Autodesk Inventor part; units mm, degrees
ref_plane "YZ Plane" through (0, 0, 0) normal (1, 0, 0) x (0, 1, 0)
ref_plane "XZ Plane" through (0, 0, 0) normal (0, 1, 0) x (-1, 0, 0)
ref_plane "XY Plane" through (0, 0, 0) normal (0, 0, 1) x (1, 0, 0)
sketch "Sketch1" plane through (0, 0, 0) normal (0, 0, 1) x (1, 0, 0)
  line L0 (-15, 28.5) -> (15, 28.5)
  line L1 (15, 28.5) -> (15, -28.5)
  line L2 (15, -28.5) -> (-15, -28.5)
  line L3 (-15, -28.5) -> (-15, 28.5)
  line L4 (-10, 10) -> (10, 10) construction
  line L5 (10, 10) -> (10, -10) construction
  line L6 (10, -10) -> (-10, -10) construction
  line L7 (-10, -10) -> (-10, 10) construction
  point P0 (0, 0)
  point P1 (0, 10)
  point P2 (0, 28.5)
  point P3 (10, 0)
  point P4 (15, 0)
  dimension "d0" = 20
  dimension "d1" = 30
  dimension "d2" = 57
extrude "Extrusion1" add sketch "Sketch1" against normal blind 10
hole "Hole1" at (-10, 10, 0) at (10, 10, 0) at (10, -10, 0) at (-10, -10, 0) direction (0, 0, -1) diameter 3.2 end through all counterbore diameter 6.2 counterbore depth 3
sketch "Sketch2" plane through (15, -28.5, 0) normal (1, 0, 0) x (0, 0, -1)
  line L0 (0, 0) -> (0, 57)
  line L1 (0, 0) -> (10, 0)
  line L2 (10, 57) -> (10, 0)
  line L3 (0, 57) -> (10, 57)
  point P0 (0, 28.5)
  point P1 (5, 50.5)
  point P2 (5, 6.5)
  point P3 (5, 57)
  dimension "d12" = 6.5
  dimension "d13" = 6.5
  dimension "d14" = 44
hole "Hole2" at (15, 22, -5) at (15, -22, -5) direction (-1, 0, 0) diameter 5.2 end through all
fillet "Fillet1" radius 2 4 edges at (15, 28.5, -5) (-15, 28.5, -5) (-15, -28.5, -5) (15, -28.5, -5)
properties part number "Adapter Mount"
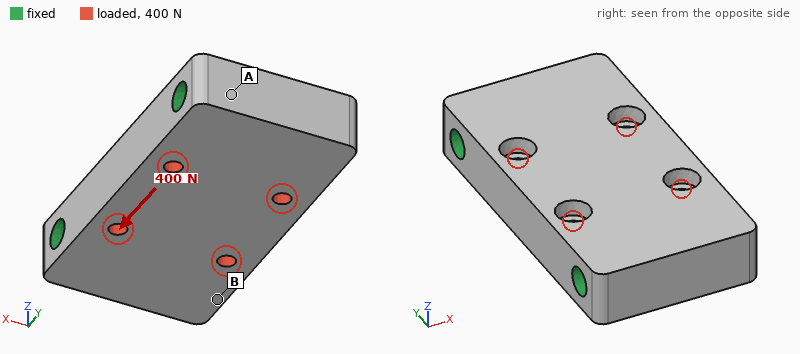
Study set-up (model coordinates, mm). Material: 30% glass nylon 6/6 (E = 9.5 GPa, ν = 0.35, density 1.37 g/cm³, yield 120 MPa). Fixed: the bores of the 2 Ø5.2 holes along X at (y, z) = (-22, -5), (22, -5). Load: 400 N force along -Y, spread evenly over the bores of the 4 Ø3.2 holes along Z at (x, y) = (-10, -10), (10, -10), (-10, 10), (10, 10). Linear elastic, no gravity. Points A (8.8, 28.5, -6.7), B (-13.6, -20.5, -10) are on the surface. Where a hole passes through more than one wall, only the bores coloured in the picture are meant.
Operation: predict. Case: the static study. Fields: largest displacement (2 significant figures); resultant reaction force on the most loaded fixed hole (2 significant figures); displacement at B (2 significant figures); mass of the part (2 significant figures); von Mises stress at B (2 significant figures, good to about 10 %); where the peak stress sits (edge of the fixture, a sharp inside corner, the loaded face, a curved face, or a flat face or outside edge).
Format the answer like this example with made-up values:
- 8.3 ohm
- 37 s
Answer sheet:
- 1.5 µm
- 200 N
- 0.27 µm
- 21 g
- 0.49 MPa
- the loaded face
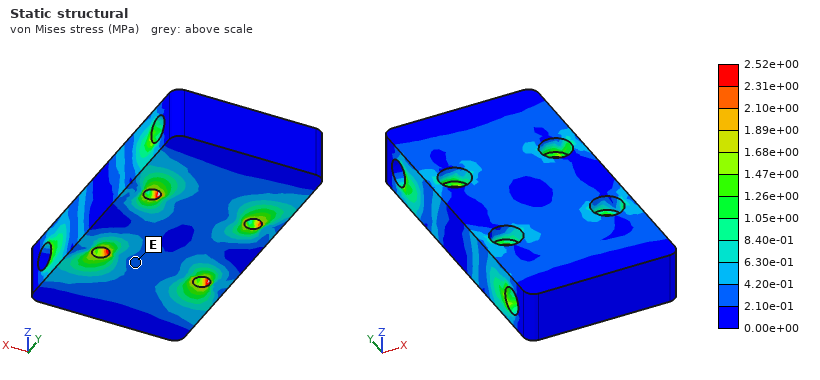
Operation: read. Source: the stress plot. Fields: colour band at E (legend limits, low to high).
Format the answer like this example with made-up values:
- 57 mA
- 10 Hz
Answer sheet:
- 2.10e-01 to 4.20e-01 MPa
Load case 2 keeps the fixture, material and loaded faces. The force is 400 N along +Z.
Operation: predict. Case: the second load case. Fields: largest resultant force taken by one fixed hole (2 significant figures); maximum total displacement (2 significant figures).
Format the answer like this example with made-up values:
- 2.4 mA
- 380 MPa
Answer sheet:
- 200 N
- 8.0 µm
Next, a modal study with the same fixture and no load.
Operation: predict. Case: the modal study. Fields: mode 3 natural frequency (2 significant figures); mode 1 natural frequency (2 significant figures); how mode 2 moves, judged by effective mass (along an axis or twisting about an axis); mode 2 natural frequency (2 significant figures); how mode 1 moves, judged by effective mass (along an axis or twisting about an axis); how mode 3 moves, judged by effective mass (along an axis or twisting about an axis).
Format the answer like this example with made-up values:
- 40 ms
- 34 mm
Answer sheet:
- 17 kHz
- 11 kHz
- twisting about Y
- 14 kHz
- along Z
- along X
